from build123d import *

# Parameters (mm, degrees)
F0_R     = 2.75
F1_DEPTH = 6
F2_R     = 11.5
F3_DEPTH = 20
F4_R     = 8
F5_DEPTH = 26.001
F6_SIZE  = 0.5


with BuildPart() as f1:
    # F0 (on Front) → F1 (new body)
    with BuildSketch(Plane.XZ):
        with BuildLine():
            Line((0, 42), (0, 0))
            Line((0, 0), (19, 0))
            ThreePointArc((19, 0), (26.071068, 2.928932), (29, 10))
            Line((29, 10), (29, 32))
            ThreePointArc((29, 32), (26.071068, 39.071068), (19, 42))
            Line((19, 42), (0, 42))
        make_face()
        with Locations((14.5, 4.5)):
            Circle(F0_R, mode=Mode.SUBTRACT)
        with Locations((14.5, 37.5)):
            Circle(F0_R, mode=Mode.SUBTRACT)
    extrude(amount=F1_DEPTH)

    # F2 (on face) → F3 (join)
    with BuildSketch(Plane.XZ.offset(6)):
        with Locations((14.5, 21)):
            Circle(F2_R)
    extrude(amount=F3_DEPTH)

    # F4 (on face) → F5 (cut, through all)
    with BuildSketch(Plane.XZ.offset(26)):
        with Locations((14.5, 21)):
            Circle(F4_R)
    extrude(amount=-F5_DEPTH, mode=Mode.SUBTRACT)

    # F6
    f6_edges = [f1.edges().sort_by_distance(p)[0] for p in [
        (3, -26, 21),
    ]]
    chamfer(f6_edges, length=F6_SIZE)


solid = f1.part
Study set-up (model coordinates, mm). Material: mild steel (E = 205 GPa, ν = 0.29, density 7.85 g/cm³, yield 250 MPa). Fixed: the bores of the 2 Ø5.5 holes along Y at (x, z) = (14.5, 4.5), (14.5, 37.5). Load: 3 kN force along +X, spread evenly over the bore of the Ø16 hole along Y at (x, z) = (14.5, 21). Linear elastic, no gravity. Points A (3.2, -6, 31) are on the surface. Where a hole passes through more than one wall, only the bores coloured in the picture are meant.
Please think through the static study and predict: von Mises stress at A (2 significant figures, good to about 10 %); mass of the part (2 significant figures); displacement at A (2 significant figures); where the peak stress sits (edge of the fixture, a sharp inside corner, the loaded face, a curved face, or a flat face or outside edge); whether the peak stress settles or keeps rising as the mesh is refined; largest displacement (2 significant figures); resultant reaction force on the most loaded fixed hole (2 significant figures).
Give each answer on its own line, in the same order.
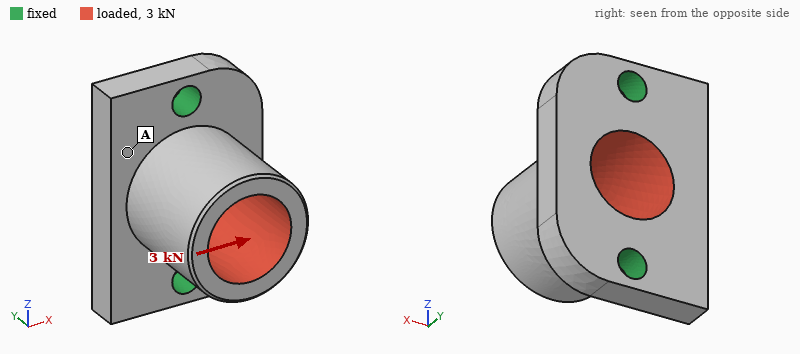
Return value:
24 MPa
77 g
9.0 µm
edge of the fixture
keeps rising
29 µm
1.5 kN
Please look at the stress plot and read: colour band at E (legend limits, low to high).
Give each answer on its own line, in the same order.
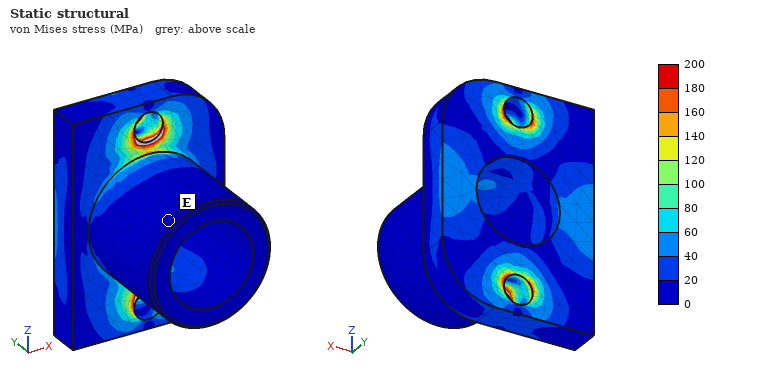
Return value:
0 to 20 MPa
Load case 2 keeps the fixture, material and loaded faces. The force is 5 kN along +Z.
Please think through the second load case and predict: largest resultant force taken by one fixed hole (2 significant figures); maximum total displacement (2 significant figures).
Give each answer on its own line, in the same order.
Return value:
3.1 kN
12 µm
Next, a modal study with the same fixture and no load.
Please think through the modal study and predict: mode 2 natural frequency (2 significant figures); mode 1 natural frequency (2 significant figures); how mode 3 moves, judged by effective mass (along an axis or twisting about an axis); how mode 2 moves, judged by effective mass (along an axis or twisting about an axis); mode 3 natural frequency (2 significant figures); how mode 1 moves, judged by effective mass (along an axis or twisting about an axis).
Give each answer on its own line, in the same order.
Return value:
18 kHz
8200 Hz
along Y
along Z
19 kHz
along X
